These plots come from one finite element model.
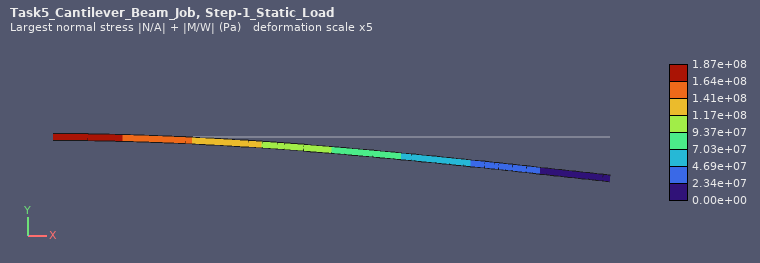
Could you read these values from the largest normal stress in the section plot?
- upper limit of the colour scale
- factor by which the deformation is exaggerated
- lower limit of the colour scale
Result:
1.87e+08 Pa
5
0.00e+00 Pa
